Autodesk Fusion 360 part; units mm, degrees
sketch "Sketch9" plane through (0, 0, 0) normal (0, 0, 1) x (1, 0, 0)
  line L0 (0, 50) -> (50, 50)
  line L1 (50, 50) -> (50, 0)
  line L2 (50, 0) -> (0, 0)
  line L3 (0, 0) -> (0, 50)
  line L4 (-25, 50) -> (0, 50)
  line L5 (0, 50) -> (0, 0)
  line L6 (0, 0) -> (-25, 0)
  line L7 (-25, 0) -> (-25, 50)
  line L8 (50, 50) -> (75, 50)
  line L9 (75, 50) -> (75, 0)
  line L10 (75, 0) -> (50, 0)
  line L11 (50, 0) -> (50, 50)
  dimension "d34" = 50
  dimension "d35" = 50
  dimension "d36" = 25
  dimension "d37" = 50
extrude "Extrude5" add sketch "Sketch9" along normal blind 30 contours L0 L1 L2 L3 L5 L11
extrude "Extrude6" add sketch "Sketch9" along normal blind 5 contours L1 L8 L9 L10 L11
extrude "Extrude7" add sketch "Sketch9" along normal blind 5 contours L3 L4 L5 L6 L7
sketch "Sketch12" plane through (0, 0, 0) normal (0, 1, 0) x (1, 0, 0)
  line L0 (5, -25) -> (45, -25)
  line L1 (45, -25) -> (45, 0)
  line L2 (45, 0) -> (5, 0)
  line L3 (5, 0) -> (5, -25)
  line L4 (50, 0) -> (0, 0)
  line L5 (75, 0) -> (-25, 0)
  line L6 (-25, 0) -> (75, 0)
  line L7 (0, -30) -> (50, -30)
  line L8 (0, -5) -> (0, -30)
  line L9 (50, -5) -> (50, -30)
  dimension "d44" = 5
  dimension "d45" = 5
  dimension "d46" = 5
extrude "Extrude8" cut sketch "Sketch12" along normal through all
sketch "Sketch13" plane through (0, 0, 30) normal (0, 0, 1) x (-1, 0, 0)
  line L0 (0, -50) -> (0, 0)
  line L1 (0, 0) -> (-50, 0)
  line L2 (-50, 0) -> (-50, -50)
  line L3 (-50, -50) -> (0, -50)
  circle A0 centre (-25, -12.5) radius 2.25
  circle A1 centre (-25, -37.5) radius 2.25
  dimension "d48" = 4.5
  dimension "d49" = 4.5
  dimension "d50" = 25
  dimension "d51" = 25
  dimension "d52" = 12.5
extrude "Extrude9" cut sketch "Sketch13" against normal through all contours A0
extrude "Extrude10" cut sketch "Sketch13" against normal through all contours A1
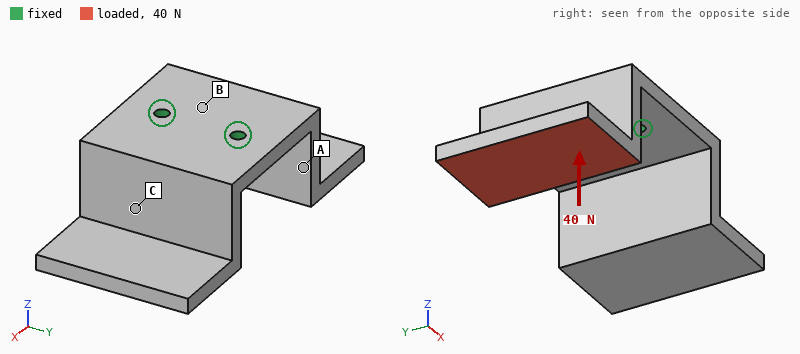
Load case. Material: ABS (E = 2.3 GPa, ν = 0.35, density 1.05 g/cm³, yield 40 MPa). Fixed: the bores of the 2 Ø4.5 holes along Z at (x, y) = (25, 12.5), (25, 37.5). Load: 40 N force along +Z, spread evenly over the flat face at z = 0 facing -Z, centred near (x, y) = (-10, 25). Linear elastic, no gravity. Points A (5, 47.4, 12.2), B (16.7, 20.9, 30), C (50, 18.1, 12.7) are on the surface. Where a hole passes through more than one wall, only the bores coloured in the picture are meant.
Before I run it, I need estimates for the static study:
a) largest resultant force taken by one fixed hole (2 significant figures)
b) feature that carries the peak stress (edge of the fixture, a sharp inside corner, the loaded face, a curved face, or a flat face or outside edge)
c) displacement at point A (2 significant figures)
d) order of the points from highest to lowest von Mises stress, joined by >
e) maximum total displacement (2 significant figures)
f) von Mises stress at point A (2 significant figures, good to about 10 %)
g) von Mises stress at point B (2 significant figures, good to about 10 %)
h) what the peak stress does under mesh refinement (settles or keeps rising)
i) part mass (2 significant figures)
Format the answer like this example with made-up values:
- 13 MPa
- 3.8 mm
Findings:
- 20 N
- edge of the fixture
- 0.35 mm
- B > A > C
- 1.2 mm
- 2.2 MPa
- 4.3 MPa
- keeps rising
- 39 g
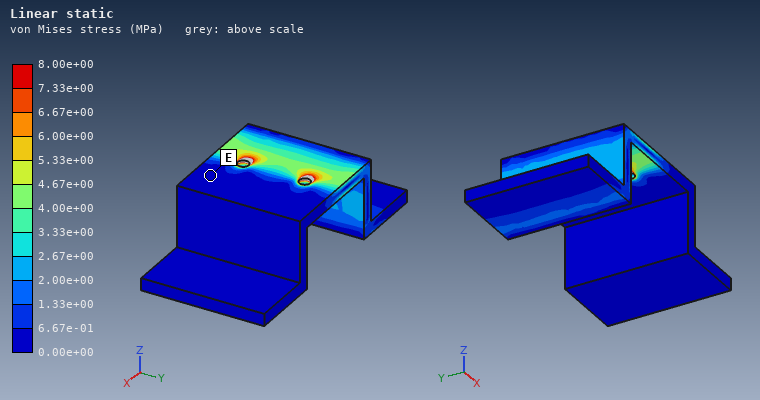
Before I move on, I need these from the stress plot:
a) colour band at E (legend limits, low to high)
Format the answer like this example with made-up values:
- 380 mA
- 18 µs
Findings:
- 0.00e+00 to 6.67e-01 MPa
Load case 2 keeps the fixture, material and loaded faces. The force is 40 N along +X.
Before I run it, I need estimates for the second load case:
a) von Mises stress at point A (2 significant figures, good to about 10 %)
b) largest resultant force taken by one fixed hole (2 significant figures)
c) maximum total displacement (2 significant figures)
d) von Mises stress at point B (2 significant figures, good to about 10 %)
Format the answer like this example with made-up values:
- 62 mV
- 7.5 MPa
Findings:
- 2.3 MPa
- 21 N
- 1.3 mm
- 4.3 MPa
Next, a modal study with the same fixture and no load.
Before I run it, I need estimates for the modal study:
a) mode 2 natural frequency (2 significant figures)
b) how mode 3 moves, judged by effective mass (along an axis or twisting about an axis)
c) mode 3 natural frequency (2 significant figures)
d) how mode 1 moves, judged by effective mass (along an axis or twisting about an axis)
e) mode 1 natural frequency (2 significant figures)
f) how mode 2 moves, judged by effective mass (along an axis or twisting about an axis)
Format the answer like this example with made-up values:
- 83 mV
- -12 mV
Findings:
- 320 Hz
- twisting about Z
- 700 Hz
- along X
- 290 Hz
- along Z
